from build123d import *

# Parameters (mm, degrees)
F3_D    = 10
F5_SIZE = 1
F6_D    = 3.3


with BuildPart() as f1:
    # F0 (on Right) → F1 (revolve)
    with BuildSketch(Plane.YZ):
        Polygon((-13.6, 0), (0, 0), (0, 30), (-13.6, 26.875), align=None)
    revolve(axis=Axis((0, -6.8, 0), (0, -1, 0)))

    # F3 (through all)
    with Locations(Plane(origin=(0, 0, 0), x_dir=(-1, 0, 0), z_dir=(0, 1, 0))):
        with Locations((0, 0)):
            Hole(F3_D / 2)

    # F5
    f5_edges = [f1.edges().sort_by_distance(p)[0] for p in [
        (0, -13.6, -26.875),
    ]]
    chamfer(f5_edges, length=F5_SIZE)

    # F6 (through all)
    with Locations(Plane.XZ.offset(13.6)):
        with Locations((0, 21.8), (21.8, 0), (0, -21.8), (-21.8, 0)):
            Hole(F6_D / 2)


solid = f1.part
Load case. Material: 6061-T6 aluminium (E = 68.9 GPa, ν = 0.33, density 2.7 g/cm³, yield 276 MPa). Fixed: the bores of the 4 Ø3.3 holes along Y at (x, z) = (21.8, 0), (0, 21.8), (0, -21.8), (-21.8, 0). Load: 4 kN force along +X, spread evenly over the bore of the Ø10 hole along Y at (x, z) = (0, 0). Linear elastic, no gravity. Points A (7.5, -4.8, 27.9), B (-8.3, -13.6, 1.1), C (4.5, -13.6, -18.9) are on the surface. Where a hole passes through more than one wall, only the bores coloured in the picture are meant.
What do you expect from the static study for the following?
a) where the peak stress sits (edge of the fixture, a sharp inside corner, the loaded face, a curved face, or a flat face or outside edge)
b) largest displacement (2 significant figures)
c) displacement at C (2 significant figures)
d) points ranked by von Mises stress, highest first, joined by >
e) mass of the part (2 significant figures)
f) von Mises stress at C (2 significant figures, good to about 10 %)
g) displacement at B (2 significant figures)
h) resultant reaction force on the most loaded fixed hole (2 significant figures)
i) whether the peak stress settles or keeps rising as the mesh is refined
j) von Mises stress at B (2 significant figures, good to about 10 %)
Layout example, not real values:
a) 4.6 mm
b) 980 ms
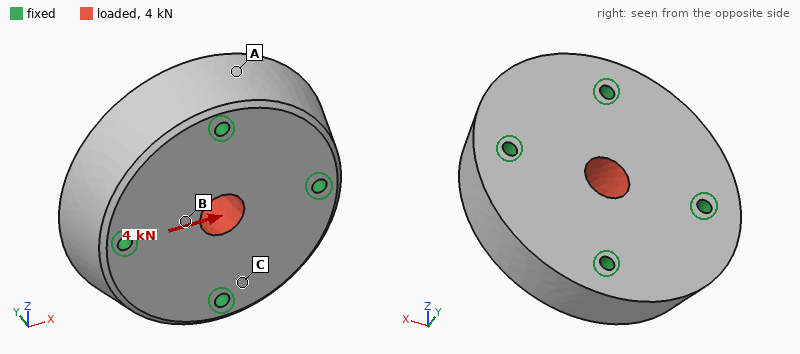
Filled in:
a) edge of the fixture
b) 2.4 µm
c) 0.45 µm
d) B > C > A
e) 89 g
f) 3.2 MPa
g) 1.8 µm
h) 1.3 kN
i) keeps rising
j) 9.9 MPa
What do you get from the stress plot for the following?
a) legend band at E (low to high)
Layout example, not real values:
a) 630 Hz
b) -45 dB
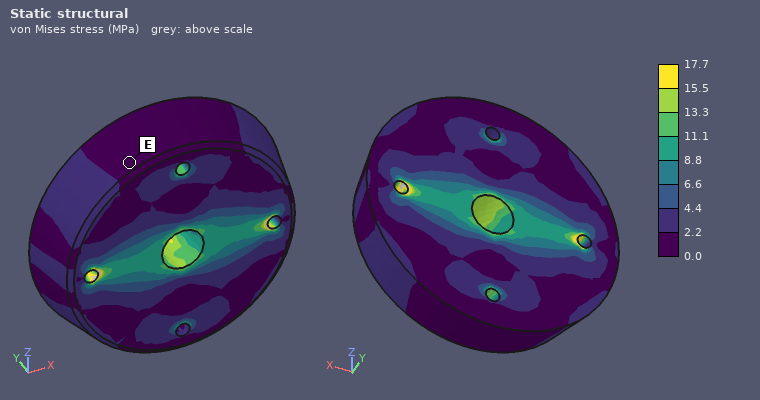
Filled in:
a) 0.0 to 2.2 MPa
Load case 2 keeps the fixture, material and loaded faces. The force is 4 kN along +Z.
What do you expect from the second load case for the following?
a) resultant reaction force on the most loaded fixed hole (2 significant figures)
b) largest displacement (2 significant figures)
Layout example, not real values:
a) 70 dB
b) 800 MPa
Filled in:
a) 1.3 kN
b) 2.4 µm
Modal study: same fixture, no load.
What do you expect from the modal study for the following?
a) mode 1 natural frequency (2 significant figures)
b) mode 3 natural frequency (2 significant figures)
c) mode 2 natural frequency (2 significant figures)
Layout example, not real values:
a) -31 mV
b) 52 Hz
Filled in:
a) 29 kHz
b) 30 kHz
c) 29 kHz
